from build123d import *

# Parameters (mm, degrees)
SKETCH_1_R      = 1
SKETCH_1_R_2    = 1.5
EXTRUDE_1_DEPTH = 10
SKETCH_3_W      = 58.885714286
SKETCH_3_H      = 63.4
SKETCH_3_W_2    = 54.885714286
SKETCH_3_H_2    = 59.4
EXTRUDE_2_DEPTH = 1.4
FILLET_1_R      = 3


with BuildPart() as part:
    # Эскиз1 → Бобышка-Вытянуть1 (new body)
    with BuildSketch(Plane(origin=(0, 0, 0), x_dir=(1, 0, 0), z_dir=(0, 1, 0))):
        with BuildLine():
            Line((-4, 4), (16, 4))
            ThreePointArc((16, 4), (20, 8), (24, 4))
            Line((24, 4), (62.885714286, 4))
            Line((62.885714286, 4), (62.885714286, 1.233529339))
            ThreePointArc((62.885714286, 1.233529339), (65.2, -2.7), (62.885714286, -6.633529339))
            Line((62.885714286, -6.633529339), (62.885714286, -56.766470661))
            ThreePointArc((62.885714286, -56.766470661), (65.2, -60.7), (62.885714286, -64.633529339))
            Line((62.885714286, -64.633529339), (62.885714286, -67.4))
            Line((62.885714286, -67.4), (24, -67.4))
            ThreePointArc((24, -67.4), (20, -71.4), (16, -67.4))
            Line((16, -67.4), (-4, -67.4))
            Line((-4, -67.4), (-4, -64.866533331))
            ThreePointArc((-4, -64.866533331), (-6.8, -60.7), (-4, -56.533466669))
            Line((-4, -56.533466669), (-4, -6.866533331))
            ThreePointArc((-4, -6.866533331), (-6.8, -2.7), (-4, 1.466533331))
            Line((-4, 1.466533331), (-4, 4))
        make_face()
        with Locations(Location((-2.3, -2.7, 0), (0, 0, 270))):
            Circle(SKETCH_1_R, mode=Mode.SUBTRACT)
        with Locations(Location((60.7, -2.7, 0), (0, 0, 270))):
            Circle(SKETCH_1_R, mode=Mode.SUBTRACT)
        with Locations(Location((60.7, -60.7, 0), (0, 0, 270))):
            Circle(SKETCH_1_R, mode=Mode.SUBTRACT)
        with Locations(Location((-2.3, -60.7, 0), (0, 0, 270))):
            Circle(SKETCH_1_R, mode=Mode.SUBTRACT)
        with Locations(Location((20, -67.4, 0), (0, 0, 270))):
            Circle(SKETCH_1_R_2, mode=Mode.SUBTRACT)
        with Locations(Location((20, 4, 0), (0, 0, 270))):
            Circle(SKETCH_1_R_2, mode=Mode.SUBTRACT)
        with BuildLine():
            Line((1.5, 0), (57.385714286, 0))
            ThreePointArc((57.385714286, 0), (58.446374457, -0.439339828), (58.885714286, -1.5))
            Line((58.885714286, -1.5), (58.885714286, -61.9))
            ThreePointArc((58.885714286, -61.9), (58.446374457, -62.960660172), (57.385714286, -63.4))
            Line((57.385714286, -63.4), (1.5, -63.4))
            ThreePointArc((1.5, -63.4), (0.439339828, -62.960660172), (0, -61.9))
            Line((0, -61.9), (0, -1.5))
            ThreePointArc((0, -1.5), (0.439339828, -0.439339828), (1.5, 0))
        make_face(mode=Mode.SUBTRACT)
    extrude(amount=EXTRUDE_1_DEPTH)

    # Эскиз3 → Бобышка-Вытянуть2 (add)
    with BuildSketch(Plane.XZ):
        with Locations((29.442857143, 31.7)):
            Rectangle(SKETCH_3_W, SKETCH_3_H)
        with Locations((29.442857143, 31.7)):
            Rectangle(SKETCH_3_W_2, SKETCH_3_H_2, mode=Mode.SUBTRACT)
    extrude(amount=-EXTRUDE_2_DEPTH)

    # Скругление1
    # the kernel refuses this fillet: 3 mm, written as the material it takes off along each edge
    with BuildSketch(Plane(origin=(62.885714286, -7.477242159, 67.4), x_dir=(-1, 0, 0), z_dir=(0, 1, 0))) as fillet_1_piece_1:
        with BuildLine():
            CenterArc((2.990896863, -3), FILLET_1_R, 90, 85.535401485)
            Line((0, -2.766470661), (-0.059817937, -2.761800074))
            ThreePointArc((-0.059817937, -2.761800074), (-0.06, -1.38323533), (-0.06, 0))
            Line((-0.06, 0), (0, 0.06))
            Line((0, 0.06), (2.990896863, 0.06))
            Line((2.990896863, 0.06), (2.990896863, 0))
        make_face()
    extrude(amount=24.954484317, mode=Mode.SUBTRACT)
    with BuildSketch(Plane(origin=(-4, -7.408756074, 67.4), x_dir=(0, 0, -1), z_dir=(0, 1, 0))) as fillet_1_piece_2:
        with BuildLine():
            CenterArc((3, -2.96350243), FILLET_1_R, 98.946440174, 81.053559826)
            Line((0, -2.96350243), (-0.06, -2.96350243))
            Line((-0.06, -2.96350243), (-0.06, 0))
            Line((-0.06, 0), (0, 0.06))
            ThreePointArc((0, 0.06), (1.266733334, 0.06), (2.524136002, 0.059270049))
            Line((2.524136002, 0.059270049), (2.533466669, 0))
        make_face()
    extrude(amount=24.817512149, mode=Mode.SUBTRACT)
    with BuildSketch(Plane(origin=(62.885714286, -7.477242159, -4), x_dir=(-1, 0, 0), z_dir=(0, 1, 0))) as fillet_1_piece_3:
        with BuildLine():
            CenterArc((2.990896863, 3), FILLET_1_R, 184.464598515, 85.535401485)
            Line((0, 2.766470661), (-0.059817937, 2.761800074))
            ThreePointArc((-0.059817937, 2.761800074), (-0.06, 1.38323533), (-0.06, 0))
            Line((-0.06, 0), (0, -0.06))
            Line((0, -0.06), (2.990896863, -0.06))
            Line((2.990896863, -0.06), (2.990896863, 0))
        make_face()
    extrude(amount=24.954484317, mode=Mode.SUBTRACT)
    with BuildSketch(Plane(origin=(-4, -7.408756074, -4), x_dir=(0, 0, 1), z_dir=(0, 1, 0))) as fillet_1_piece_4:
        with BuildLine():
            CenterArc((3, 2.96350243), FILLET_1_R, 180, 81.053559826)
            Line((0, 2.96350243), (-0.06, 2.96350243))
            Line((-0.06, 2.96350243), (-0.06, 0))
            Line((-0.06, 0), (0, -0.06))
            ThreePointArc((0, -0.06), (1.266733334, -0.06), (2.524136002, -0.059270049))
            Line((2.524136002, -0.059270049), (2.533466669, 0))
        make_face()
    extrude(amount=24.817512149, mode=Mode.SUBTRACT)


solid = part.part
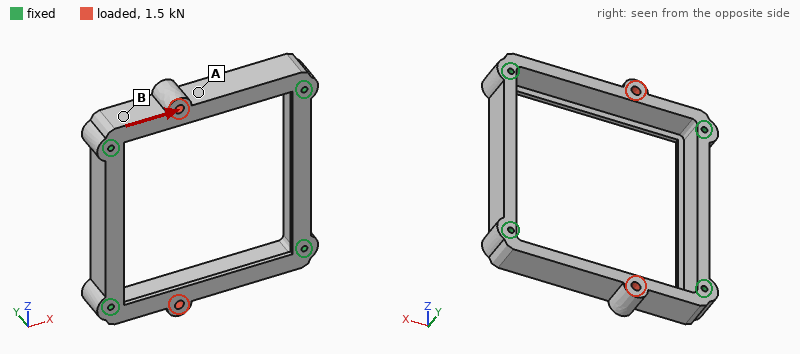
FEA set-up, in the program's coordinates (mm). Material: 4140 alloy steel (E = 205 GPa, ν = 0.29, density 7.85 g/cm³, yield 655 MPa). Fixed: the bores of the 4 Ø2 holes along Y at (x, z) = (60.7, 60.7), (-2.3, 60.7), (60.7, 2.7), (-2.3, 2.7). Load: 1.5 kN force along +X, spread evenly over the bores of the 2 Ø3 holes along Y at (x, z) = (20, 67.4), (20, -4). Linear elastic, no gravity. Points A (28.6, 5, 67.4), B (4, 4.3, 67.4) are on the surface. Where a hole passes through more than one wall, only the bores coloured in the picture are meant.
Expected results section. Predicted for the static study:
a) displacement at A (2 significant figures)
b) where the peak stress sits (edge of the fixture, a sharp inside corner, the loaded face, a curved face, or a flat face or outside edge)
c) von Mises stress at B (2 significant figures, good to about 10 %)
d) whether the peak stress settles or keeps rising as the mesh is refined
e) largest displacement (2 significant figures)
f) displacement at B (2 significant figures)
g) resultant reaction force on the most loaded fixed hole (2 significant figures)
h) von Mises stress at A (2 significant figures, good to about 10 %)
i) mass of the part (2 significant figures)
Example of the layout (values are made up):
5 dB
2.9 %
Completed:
6.2 µm
edge of the fixture
7.5 MPa
keeps rising
6.5 µm
1.9 µm
420 N
26 MPa
93 g
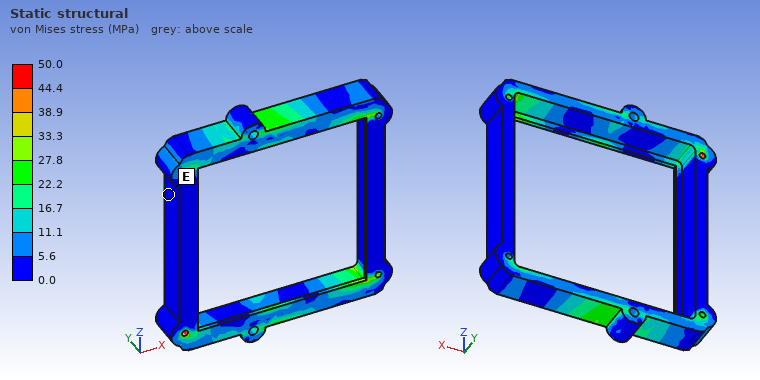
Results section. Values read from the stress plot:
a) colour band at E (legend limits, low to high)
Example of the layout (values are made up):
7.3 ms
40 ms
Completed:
0.0 to 5.6 MPa
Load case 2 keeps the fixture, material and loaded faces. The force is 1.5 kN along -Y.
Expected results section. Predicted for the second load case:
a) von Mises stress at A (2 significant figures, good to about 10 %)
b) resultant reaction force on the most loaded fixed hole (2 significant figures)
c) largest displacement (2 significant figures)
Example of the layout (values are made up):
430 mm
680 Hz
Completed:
30 MPa
520 N
26 µm
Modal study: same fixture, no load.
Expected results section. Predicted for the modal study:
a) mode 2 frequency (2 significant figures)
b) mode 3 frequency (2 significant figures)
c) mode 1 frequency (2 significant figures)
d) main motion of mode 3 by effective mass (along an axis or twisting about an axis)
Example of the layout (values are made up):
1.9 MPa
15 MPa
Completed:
5500 Hz
7000 Hz
5500 Hz
along X
